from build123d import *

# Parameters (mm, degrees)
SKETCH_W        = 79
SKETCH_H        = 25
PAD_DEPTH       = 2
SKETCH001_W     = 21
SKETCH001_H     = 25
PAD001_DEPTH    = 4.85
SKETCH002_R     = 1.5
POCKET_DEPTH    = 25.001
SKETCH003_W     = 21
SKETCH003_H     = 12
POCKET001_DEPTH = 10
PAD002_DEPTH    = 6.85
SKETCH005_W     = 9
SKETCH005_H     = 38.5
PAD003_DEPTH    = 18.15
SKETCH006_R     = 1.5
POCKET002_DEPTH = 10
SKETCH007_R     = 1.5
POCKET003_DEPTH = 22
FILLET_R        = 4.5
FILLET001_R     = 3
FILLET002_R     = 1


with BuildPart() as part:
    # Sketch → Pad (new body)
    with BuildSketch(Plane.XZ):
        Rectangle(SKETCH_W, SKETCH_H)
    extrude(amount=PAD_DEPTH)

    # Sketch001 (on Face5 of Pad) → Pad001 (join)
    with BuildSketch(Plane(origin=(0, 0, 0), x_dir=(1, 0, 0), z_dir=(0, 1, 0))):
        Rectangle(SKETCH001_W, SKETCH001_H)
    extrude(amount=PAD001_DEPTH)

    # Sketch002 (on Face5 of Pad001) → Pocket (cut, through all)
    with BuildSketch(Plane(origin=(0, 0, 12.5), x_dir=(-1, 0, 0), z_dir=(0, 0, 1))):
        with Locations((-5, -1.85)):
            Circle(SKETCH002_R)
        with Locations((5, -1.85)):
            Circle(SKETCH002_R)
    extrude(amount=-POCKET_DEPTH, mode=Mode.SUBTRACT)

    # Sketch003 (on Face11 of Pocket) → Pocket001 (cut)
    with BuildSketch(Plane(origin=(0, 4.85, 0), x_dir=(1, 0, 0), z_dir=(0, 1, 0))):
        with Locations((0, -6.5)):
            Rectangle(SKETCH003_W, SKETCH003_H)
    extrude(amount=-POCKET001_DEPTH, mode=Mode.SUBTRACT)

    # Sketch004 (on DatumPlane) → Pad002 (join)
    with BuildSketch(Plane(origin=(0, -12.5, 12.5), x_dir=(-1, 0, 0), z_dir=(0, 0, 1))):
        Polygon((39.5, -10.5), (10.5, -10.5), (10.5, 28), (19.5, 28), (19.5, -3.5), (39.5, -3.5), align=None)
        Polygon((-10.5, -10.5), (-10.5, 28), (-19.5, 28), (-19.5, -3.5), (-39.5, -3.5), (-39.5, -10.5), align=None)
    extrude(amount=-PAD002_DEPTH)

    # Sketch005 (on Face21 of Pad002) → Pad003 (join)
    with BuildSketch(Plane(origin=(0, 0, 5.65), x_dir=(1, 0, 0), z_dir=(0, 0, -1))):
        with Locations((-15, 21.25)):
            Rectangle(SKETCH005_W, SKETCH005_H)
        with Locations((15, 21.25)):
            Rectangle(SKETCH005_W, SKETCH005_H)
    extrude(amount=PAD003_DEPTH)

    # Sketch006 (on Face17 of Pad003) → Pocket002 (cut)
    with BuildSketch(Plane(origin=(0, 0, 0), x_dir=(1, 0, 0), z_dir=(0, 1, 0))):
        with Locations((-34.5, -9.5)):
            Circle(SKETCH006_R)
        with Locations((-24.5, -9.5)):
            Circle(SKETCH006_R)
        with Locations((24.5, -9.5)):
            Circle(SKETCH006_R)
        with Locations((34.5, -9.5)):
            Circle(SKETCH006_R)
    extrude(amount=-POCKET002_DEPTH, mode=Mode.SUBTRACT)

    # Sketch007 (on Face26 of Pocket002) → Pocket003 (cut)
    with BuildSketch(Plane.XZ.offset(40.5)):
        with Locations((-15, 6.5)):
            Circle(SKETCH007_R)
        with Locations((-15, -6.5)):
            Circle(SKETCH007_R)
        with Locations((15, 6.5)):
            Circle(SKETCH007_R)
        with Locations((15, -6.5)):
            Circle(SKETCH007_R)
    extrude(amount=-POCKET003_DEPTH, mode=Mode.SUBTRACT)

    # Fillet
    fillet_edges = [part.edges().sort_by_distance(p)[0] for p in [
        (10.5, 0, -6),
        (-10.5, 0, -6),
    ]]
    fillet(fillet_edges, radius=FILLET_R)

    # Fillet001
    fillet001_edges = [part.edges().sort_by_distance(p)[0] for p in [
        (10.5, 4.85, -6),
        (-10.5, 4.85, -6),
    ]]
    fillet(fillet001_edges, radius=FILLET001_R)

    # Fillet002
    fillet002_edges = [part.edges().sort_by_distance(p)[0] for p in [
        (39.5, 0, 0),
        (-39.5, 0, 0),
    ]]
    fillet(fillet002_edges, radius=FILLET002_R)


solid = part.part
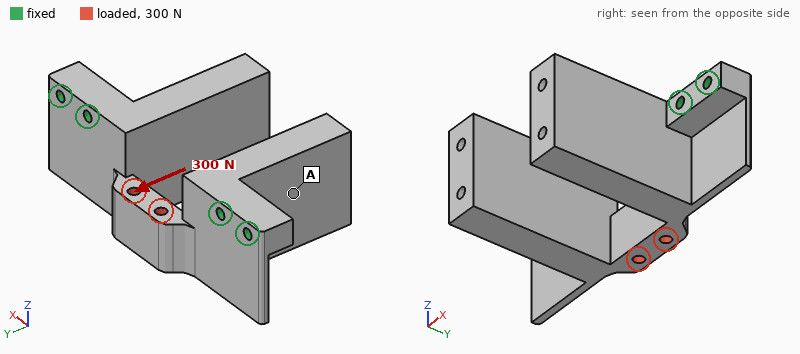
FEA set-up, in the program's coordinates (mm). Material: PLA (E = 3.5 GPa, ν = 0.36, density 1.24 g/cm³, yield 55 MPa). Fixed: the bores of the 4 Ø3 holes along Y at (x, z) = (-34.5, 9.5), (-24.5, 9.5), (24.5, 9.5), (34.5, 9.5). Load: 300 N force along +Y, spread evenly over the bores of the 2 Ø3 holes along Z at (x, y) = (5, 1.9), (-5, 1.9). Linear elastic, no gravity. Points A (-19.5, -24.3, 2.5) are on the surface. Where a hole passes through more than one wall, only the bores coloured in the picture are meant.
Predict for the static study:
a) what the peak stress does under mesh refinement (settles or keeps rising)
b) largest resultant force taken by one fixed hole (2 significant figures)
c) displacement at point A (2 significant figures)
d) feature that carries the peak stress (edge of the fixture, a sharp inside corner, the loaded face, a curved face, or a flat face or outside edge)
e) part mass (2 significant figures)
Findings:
keeps rising
170 N
0.34 mm
edge of the fixture
29 g
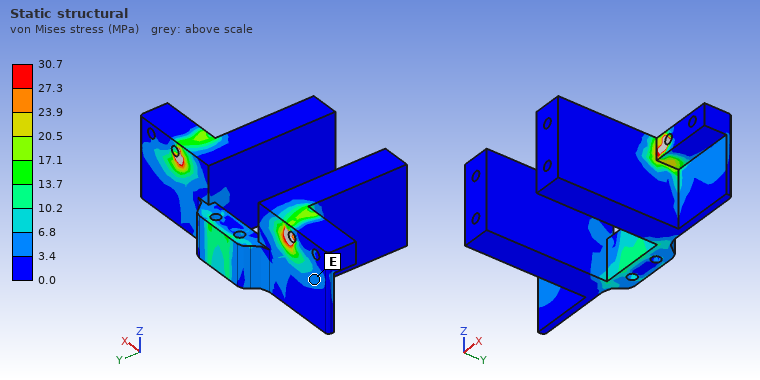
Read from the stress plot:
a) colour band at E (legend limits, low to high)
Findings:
3.4 to 6.8 MPa
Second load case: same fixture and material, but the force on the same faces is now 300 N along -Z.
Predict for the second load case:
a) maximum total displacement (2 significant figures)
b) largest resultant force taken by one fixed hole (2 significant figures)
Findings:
0.26 mm
190 N
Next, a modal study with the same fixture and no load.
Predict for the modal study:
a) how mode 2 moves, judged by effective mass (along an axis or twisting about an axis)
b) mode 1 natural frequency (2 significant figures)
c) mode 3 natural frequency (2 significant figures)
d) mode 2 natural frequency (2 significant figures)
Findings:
along X
770 Hz
940 Hz
880 Hz
